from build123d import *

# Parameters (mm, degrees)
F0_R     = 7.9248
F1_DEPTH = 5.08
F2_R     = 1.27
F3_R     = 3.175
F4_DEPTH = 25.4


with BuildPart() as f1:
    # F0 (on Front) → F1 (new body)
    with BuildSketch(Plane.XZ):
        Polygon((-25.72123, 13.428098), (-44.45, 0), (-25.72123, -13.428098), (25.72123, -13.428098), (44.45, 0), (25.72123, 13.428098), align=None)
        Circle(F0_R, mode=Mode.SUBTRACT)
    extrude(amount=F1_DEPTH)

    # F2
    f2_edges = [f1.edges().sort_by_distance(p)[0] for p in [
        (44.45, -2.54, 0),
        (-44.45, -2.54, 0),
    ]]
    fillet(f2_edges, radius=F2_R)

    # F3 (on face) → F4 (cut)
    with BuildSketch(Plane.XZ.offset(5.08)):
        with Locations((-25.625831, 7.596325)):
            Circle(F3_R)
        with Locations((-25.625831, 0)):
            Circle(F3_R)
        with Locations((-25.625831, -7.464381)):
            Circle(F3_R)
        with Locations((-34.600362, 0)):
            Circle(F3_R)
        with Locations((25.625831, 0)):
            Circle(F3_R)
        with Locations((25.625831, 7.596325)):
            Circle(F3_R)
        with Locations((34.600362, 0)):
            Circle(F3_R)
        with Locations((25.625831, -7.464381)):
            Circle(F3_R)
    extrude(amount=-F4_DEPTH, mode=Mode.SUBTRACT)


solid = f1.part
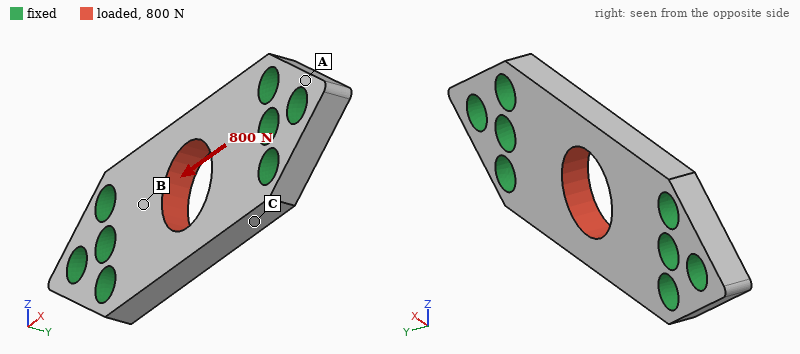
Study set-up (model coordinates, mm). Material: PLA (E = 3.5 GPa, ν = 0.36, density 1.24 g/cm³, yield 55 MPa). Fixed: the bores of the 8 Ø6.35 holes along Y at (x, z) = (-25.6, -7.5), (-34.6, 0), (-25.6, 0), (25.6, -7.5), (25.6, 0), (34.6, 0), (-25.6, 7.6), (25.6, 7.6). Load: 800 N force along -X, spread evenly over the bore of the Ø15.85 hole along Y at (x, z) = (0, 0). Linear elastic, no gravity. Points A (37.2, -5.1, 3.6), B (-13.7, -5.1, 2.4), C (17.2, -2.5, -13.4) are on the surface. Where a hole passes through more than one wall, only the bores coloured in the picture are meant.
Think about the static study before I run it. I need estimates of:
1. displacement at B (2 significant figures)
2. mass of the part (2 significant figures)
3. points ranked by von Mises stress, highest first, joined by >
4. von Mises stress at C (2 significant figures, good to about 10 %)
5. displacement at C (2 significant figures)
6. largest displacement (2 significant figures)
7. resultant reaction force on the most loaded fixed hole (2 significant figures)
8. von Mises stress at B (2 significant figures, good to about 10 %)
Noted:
8.0 µm
9.0 g
B > C > A
2.0 MPa
7.7 µm
21 µm
150 N
3.5 MPa
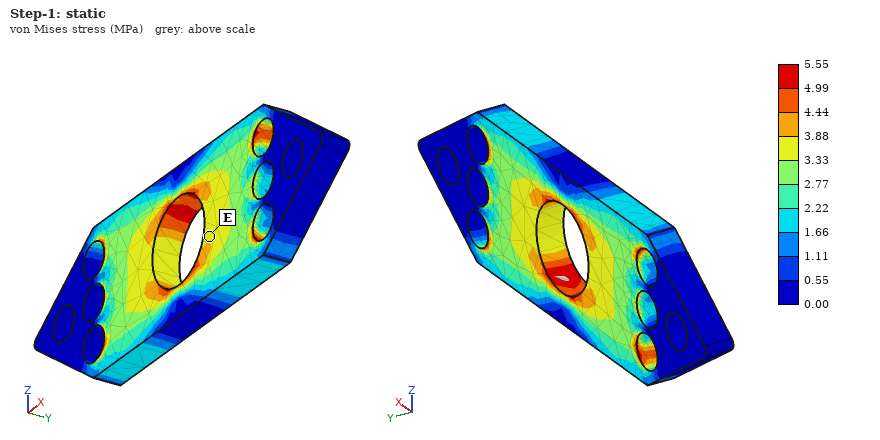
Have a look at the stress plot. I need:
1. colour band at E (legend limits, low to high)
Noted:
3.33 to 3.88 MPa
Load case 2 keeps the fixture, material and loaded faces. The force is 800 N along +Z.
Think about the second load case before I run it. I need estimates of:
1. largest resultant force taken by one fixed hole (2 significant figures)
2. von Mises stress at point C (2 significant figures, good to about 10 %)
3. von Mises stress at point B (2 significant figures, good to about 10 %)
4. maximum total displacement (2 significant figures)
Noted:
240 N
3.0 MPa
8.0 MPa
79 µm
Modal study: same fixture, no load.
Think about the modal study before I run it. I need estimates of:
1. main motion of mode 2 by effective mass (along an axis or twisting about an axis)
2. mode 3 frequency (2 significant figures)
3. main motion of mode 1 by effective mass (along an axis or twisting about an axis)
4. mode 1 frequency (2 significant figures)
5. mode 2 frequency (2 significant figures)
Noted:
twisting about X
9000 Hz
along Y
4300 Hz
5200 Hz
